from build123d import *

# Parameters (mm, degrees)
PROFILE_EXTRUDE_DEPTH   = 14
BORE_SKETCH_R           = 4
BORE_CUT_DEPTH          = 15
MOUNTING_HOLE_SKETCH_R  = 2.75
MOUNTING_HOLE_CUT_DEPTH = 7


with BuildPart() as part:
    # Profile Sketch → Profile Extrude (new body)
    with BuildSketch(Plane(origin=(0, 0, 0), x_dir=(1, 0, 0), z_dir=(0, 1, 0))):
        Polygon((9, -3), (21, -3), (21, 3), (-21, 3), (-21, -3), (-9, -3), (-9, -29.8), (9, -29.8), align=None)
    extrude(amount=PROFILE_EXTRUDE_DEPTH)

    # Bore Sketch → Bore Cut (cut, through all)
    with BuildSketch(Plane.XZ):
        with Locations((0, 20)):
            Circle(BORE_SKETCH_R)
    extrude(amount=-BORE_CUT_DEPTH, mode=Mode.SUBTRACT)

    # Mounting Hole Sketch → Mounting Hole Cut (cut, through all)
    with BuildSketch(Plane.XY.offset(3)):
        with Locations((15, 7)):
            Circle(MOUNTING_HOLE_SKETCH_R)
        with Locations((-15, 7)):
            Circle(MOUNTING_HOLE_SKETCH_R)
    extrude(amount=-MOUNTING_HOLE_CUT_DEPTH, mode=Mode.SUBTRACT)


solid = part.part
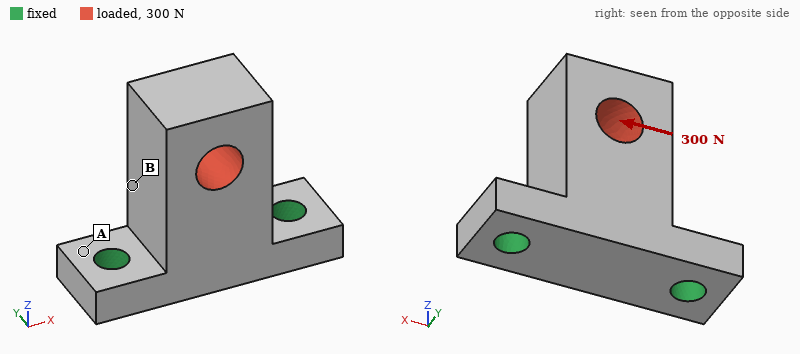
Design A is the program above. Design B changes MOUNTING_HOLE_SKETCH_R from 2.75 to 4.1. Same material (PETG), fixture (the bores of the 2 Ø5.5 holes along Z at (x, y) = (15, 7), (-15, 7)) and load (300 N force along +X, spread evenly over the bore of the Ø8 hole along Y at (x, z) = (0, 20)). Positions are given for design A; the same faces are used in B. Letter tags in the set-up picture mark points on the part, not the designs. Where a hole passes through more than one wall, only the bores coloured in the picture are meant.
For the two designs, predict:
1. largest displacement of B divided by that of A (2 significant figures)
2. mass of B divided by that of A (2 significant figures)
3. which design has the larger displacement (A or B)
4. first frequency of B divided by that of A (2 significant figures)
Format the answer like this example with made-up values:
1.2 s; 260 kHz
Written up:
0.86; 0.96; A; 1.2
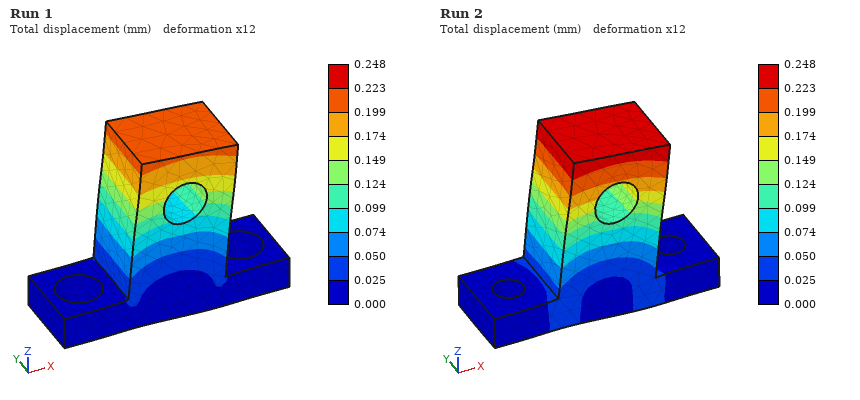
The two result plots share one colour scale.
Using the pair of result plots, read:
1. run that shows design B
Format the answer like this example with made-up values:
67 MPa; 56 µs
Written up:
Run 1
